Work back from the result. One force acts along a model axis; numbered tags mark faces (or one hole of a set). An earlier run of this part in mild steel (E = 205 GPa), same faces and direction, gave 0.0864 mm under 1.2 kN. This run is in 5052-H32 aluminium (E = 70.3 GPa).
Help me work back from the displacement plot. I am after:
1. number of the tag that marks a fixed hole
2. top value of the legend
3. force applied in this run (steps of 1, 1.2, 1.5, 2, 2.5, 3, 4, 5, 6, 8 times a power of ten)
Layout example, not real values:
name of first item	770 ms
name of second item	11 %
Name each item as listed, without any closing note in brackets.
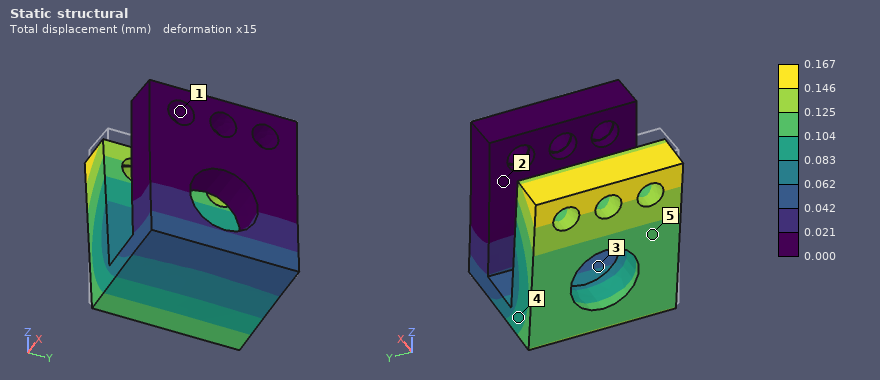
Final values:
number of the tag that marks a fixed hole	1
top value of the legend	0.167 mm
force applied in this run	800 N
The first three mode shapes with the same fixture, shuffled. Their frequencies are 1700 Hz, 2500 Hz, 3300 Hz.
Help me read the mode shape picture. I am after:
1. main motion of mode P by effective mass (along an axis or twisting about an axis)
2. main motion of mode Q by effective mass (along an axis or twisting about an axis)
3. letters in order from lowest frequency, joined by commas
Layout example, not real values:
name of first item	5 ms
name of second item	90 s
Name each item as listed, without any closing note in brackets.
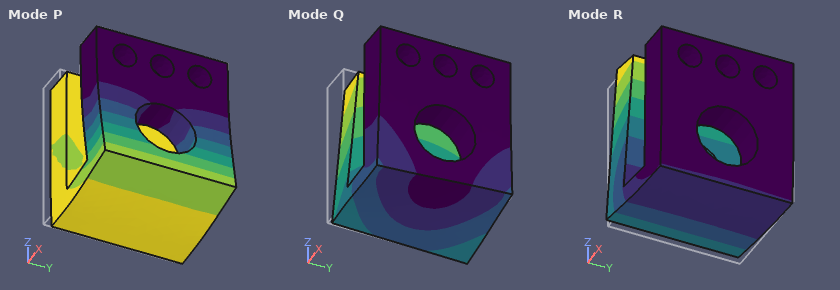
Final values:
main motion of mode P by effective mass	along X
main motion of mode Q by effective mass	along Y
letters in order from lowest frequency, joined by commas	R, Q, P
